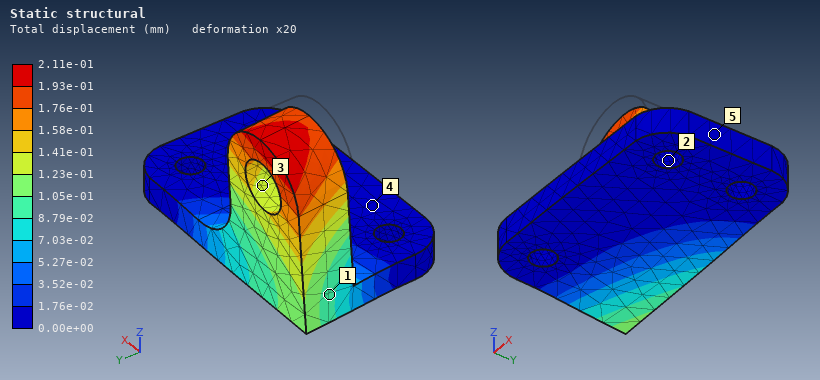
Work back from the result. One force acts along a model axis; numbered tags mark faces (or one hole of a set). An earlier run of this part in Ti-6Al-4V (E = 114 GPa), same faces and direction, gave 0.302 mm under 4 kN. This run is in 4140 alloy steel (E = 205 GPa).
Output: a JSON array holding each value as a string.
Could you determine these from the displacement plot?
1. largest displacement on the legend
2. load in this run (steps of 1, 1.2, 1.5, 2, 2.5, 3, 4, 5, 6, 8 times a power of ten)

["2.11e-01 mm", "5 kN"]
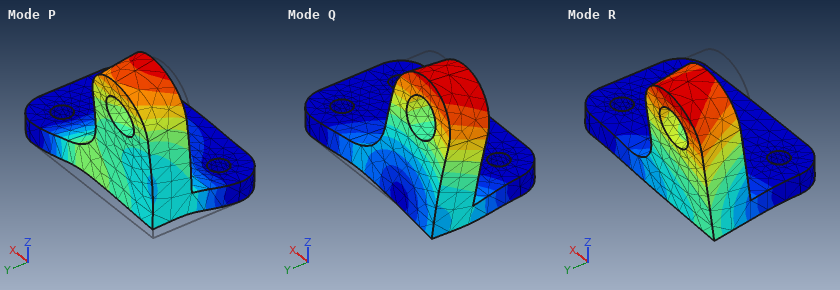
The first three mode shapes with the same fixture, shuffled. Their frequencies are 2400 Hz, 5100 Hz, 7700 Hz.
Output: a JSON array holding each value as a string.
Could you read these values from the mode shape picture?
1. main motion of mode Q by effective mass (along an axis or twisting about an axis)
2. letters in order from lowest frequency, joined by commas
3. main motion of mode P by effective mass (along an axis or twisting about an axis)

["along X", "R, Q, P", "along Z"]
